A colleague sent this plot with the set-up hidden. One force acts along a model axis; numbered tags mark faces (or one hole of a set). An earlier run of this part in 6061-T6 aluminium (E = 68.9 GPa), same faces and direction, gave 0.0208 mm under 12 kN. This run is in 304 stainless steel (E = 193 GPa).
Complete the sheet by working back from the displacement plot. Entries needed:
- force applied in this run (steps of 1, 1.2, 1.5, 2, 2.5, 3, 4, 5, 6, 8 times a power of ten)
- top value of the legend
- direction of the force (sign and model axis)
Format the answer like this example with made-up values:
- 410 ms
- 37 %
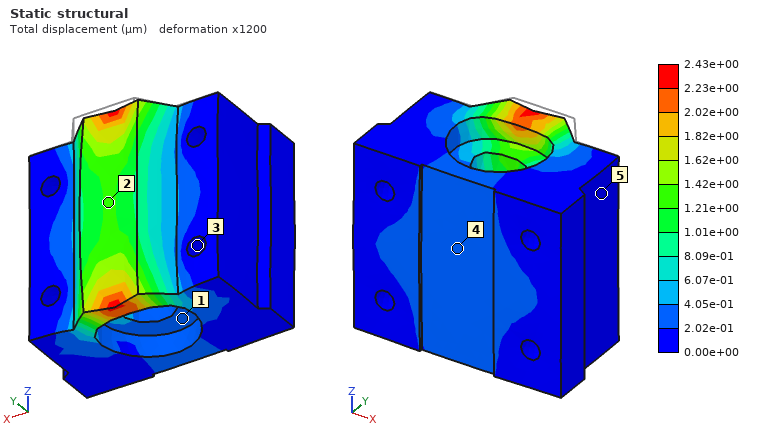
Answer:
- 4 kN
- 2.43e+00 µm
- -Y
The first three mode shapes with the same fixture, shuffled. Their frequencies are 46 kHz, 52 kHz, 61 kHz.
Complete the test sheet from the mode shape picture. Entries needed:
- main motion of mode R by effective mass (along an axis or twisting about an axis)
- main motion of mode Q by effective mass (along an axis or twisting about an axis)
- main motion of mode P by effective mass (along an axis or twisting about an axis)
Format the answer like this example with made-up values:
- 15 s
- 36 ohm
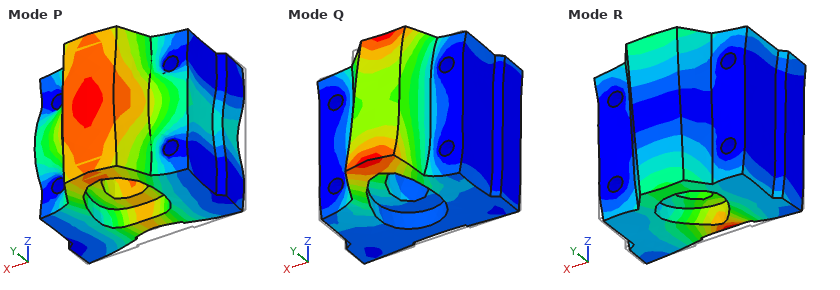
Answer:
- along Z
- along Z
- along Y
